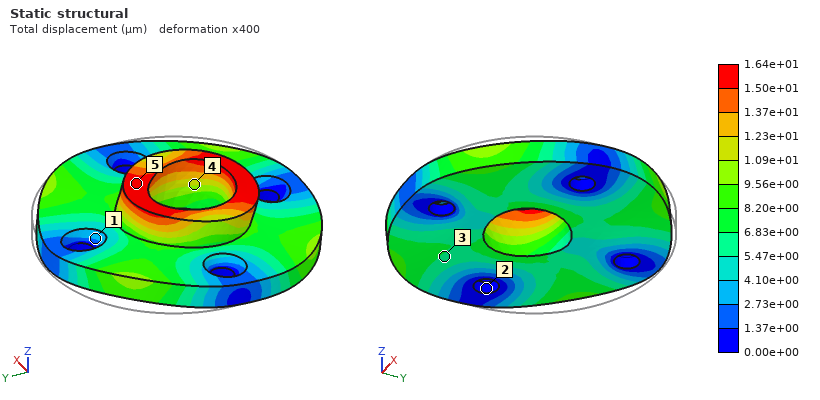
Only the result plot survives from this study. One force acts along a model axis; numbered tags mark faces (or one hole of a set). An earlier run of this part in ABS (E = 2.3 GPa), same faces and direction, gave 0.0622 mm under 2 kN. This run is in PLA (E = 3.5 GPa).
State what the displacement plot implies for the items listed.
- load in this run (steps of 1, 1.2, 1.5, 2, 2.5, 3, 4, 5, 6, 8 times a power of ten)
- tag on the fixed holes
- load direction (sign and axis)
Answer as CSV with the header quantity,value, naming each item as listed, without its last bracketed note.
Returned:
quantity,value
load in this run,800 N
tag on the fixed holes,2
load direction,-Y
